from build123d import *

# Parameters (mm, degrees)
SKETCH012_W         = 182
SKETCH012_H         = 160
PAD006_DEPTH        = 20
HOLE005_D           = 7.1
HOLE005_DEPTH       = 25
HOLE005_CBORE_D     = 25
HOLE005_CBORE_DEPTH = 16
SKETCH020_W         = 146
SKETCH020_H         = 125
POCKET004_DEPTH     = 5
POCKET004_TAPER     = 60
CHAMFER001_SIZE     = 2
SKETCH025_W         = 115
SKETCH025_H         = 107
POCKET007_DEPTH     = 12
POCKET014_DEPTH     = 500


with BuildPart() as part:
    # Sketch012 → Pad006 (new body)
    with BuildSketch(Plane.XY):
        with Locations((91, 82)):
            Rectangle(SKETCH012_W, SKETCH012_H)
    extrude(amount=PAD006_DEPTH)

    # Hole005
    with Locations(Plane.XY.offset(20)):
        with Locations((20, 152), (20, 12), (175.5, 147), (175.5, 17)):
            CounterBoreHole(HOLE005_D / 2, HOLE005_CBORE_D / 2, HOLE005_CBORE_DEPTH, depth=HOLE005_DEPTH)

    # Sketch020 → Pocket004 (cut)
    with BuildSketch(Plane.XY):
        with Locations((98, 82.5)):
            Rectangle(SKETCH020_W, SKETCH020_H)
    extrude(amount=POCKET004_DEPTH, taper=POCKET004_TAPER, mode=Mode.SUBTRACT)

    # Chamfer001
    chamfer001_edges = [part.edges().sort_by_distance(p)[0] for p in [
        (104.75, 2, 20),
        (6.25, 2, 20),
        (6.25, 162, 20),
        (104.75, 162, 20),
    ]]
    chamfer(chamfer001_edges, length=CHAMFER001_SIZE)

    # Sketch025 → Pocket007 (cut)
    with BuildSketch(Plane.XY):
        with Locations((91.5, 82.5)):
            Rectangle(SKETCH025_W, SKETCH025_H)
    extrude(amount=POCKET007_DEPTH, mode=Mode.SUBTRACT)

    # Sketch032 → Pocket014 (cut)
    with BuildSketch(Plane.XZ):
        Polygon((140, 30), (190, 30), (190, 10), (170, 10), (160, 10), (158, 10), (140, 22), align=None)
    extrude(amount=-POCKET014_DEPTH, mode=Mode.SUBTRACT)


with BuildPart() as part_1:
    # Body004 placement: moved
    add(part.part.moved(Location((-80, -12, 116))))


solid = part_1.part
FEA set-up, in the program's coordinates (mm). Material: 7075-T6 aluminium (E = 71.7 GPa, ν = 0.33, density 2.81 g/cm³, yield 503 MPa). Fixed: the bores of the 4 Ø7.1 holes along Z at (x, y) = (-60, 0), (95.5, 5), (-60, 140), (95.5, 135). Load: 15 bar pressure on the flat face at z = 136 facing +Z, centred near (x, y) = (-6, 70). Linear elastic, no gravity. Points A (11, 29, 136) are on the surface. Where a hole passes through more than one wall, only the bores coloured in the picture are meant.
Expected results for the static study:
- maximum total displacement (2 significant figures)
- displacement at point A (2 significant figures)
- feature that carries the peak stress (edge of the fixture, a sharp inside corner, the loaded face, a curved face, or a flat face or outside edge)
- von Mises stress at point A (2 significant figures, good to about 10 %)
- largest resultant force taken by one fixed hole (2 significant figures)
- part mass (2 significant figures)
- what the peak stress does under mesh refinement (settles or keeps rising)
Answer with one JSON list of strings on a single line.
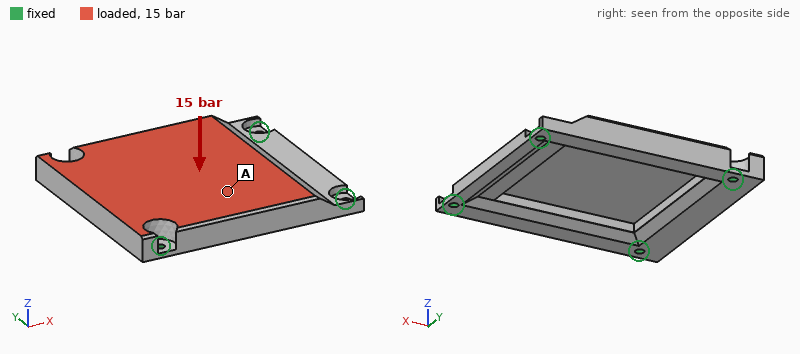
["0.50 mm", "0.37 mm", "edge of the fixture", "60 MPa", "19 kN", "970 g", "keeps rising"]
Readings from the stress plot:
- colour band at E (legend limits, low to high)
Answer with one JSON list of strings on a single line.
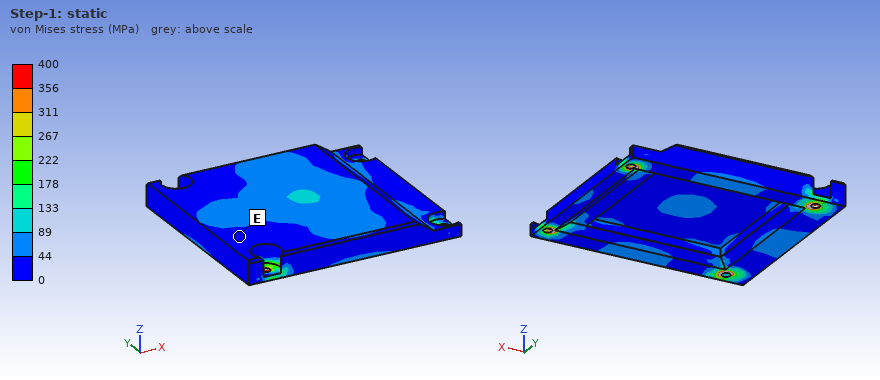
["0 to 44 MPa"]
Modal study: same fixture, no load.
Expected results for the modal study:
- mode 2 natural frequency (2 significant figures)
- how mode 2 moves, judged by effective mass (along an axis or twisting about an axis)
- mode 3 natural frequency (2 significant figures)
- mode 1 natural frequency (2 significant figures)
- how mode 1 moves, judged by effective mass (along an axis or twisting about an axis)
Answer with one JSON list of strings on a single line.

["2500 Hz", "twisting about X", "2600 Hz", "1900 Hz", "along Z"]
